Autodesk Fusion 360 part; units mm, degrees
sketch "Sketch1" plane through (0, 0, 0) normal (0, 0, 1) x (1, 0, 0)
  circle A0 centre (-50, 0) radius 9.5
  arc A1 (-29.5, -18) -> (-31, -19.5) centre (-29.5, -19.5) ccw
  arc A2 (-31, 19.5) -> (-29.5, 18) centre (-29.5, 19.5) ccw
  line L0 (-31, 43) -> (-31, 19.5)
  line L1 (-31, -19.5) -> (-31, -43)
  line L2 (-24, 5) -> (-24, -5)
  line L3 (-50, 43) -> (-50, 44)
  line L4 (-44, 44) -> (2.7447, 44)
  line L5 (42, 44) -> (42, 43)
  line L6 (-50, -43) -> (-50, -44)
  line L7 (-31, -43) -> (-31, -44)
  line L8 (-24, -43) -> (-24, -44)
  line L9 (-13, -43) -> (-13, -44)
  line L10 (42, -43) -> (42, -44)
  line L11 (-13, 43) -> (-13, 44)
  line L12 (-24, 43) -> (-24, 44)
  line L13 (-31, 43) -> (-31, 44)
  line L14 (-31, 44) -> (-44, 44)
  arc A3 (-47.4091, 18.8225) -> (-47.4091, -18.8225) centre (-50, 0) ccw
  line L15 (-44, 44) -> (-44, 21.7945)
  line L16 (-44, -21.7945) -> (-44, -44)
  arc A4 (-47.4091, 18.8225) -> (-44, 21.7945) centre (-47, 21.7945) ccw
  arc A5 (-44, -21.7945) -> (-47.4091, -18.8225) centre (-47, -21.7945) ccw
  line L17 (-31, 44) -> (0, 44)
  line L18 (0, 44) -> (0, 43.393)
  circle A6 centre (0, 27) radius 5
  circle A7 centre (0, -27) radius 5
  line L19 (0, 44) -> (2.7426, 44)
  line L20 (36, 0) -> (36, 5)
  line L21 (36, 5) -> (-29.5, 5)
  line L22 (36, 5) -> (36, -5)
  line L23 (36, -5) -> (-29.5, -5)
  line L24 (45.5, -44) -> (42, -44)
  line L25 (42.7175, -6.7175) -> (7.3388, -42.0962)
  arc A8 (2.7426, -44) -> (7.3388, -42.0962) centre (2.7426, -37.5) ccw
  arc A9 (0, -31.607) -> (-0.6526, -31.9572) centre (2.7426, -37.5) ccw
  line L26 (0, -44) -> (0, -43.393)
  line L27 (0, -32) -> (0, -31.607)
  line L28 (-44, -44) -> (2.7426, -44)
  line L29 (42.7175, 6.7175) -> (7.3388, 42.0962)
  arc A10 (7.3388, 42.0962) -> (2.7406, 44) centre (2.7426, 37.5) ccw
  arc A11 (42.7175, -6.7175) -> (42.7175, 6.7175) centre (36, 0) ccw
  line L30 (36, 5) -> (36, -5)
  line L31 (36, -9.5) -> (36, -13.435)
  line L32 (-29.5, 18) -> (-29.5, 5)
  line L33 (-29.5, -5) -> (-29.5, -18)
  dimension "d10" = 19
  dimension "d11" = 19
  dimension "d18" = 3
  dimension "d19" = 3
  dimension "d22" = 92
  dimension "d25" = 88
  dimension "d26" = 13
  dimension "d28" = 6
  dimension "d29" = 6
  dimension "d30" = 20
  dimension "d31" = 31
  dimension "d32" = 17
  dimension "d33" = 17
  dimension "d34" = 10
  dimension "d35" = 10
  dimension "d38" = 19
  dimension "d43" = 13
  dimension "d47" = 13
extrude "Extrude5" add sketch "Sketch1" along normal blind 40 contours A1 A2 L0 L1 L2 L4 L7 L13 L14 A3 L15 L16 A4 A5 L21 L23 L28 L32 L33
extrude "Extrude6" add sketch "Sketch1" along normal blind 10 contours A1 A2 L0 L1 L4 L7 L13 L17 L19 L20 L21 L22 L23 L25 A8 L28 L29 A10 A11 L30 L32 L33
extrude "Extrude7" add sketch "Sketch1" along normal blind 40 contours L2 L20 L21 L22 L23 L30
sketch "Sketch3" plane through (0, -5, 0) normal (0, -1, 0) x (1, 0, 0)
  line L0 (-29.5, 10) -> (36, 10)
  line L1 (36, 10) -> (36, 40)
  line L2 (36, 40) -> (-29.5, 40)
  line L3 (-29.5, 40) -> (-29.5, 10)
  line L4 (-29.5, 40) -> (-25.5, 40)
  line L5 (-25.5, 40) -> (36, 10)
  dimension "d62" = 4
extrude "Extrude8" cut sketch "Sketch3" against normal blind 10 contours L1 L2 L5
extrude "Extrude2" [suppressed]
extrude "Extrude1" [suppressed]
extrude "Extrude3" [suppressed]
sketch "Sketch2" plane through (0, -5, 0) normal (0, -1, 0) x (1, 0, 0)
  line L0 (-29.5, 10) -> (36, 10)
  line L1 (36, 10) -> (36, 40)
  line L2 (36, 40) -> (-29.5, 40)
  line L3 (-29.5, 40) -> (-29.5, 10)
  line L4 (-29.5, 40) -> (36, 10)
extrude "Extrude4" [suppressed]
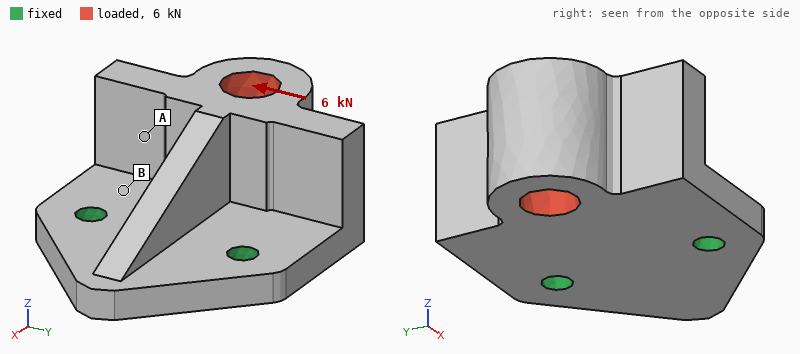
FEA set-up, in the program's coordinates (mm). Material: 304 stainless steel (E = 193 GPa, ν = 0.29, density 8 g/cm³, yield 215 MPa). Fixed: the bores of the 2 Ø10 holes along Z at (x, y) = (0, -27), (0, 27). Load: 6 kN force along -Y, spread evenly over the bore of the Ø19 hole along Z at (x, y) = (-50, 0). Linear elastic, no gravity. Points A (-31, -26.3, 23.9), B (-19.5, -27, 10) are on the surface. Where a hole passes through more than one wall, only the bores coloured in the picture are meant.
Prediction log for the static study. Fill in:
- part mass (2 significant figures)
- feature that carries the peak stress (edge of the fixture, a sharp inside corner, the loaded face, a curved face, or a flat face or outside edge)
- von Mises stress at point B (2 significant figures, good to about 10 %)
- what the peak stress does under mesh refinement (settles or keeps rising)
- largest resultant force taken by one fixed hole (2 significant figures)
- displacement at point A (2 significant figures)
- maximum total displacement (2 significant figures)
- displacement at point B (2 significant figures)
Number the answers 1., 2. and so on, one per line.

1. 1.0 kg
2. edge of the fixture
3. 28 MPa
4. keeps rising
5. 6.0 kN
6. 13 µm
7. 21 µm
8. 5.5 µm
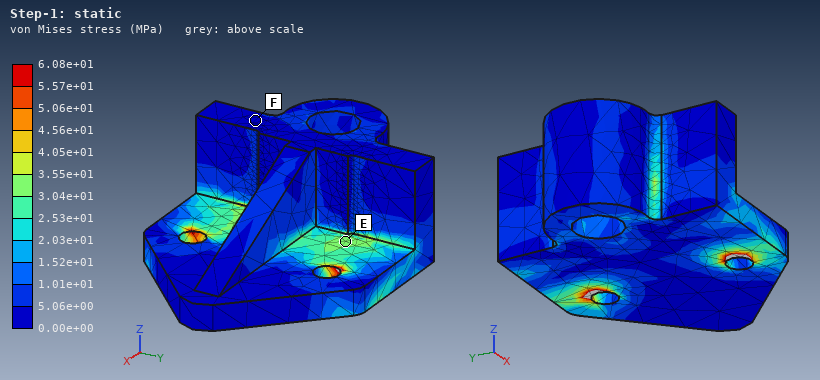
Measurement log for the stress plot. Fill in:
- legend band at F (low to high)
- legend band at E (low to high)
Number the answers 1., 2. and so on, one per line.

1. 0.00e+00 to 5.06e+00 MPa
2. 3.04e+01 to 3.55e+01 MPa
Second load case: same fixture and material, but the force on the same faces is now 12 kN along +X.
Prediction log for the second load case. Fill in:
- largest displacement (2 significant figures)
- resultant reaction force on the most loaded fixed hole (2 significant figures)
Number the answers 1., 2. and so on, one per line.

1. 0.10 mm
2. 6.0 kN
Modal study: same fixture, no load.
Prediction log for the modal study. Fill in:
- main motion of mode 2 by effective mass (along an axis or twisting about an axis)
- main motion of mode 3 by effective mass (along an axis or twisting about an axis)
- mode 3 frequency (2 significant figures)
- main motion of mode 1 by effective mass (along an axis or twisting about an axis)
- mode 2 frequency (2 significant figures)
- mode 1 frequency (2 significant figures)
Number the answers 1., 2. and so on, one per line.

1. along Y
2. along Y
3. 6400 Hz
4. along Z
5. 3500 Hz
6. 1700 Hz
